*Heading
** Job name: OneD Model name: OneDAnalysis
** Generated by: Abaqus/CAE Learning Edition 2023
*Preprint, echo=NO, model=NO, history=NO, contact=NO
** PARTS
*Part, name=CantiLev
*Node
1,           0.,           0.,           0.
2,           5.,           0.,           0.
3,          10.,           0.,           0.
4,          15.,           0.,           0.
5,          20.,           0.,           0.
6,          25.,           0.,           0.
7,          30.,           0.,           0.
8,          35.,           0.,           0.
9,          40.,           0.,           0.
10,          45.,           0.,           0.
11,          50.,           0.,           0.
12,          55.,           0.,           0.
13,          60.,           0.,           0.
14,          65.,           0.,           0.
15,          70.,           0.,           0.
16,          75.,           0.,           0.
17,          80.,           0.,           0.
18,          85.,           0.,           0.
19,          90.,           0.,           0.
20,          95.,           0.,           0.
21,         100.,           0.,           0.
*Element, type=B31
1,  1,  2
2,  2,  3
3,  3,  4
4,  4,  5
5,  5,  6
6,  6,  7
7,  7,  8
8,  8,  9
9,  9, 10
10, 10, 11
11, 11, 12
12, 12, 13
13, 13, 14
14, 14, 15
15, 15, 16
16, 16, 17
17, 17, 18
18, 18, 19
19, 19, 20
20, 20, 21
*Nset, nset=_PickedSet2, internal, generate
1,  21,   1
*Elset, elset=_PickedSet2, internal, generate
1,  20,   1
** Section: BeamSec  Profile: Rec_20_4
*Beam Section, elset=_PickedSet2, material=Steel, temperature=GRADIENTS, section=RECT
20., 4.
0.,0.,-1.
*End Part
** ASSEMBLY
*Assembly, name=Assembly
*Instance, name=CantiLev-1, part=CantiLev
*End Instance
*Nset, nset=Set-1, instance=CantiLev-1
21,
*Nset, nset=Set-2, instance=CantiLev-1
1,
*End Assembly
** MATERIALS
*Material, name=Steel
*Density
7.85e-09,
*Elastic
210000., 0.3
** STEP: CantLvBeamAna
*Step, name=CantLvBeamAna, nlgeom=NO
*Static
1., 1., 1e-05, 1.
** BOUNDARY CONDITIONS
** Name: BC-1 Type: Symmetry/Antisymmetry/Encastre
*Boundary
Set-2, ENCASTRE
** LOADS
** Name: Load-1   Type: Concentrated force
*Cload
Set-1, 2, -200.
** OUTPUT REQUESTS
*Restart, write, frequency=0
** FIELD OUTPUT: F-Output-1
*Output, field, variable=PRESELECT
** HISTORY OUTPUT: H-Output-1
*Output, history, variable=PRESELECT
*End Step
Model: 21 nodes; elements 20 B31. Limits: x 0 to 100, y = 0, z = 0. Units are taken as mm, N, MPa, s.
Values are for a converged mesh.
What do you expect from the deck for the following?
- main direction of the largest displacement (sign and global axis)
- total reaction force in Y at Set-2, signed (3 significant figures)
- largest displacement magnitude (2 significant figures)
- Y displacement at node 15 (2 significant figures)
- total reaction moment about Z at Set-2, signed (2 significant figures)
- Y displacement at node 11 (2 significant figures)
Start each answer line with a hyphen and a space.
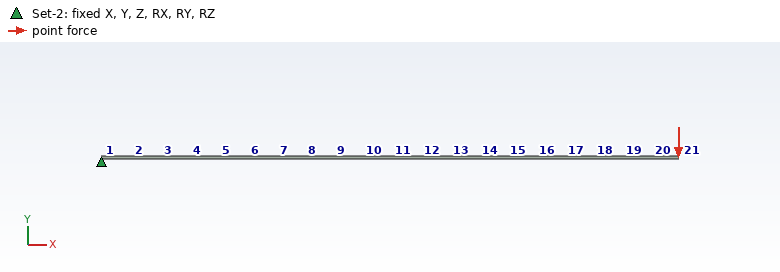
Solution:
- -Y
- 200 N
- 3.0 mm
- -1.7 mm
- 20000 N·mm
- -0.93 mm
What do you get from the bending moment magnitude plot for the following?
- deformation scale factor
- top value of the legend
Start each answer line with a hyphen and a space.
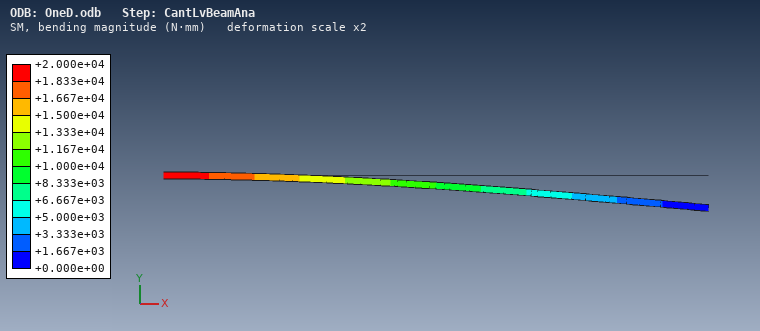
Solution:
- 2
- +2.000e+04 N·mm
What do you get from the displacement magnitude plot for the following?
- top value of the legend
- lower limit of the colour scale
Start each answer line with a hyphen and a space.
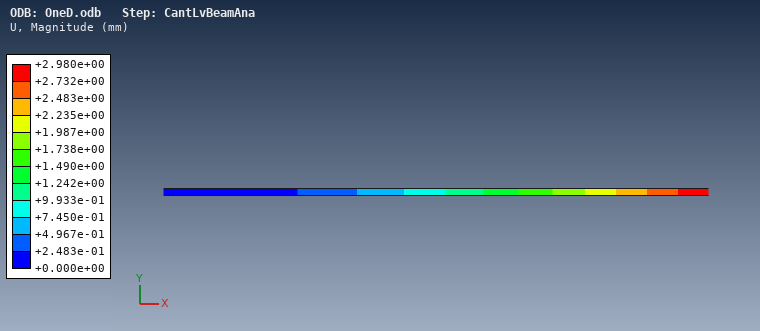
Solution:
- +2.980e+00 mm
- +0.000e+00 mm
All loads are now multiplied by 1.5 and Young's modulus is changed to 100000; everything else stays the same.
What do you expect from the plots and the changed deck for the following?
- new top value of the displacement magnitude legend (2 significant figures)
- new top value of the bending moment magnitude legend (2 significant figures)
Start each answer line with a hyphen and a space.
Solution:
- 9.4 mm
- 30000 N·mm
